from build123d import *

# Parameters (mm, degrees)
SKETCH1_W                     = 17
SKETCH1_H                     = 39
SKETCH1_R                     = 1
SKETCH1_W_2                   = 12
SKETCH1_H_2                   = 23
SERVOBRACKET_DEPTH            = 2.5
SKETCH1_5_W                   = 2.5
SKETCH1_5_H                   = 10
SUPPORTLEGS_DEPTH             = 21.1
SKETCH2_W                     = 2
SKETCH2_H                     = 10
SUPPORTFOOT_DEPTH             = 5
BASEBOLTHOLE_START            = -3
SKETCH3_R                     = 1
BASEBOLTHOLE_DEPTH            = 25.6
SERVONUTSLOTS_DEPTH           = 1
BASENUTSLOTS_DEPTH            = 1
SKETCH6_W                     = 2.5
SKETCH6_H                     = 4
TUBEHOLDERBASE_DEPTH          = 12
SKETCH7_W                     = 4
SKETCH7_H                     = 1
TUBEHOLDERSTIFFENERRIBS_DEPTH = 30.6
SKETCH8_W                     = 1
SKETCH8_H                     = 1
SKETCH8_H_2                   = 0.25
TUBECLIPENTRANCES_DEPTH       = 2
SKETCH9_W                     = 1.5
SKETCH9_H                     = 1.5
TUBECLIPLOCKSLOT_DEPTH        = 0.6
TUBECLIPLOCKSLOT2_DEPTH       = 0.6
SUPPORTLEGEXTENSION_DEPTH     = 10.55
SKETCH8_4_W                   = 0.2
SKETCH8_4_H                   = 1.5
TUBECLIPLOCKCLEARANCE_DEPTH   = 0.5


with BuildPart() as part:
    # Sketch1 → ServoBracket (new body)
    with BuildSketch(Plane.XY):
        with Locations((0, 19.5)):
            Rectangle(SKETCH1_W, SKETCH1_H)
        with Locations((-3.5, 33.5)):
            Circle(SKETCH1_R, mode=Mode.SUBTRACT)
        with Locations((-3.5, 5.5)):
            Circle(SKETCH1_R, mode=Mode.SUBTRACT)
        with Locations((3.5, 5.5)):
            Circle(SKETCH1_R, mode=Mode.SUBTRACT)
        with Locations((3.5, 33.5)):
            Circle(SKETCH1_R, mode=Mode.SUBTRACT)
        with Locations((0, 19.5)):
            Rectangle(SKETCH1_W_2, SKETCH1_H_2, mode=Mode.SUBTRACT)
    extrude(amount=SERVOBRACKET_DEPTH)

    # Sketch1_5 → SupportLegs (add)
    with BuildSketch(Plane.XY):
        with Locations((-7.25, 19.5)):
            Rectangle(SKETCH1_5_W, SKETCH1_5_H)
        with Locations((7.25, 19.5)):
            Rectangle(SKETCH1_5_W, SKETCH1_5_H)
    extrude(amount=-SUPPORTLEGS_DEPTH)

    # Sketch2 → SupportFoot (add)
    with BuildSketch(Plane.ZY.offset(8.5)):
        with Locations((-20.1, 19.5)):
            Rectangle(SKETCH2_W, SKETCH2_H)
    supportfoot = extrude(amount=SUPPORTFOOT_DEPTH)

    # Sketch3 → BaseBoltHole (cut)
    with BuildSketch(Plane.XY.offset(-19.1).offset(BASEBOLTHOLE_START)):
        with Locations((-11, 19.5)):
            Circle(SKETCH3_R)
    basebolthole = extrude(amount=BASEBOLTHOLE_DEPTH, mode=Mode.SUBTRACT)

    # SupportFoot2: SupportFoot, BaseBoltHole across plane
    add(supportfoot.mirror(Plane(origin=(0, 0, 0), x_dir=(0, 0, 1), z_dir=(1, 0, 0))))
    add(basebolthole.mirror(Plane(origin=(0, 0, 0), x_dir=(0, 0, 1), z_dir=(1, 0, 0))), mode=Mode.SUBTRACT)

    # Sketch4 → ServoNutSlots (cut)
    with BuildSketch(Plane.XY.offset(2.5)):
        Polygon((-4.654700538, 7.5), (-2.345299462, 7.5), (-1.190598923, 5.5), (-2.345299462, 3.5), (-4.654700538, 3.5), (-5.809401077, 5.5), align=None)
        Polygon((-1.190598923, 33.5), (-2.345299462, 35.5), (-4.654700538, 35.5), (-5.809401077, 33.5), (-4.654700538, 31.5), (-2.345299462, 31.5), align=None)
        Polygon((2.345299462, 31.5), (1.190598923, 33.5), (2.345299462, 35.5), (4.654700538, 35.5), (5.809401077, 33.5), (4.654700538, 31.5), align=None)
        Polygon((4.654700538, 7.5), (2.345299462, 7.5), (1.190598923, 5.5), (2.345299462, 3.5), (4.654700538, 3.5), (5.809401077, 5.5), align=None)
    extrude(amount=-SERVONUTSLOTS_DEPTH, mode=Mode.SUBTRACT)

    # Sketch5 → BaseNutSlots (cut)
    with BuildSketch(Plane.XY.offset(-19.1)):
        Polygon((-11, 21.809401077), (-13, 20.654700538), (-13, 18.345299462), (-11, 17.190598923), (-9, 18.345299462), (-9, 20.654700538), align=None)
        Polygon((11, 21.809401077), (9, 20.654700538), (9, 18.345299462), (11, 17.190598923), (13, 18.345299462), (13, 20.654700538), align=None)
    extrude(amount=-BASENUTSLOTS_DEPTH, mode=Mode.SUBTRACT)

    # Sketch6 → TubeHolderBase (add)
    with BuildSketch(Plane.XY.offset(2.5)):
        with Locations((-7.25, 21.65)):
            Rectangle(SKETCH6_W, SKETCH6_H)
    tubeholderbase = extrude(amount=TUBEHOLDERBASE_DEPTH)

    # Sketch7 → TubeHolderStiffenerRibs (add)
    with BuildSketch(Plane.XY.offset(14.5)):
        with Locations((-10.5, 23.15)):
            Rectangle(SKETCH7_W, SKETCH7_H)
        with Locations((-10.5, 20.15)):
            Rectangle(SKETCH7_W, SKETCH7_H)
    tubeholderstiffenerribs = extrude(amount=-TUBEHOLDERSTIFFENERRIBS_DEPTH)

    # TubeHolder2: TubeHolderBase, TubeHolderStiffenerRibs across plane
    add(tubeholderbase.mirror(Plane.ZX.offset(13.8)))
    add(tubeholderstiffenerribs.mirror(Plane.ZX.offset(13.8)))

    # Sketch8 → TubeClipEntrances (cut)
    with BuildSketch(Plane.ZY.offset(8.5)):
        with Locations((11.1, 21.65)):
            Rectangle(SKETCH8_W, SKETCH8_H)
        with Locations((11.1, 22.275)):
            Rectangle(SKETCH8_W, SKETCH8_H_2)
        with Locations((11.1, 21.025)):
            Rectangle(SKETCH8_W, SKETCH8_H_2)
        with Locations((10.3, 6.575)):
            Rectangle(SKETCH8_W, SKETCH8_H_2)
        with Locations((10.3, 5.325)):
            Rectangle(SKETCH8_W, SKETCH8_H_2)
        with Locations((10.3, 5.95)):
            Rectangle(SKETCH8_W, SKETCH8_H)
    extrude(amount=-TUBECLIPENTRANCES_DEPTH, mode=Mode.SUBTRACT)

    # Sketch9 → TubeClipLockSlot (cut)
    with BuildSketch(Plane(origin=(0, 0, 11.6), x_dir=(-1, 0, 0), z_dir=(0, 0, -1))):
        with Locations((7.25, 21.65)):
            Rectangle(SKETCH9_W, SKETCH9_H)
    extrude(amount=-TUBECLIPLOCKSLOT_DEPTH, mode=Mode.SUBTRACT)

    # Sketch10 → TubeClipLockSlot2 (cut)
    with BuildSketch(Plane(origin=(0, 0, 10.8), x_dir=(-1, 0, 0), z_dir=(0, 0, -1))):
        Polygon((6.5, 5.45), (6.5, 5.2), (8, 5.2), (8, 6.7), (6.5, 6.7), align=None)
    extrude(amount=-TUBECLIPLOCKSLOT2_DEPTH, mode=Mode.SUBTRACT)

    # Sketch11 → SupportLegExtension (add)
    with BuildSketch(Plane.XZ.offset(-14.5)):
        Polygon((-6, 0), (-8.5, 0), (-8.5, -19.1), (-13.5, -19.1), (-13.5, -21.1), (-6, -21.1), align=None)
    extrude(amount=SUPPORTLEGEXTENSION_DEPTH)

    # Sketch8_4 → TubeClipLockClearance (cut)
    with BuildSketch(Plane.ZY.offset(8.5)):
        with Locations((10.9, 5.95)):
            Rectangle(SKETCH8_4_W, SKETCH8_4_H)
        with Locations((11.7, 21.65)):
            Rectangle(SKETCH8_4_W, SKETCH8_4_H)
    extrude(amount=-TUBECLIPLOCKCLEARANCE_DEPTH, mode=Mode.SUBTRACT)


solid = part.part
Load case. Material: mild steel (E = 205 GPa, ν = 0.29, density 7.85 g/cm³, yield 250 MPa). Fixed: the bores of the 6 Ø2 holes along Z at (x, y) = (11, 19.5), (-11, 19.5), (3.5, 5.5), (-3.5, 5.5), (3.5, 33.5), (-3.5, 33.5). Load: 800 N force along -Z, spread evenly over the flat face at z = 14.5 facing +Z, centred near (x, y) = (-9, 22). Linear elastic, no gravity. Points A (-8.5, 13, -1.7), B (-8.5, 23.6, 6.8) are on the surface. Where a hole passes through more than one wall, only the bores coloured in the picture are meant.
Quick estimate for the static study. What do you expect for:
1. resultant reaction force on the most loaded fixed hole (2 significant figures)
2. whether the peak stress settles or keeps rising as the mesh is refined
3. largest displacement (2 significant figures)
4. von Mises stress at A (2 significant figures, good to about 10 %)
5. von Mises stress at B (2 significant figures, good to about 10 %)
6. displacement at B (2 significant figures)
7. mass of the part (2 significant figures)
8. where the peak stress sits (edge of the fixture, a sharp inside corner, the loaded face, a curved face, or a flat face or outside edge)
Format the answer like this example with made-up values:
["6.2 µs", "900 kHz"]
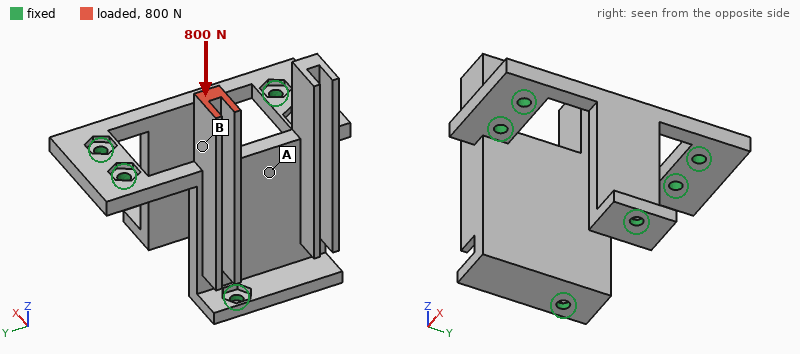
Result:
["480 N", "keeps rising", "20 µm", "21 MPa", "44 MPa", "13 µm", "27 g", "edge of the fixture"]
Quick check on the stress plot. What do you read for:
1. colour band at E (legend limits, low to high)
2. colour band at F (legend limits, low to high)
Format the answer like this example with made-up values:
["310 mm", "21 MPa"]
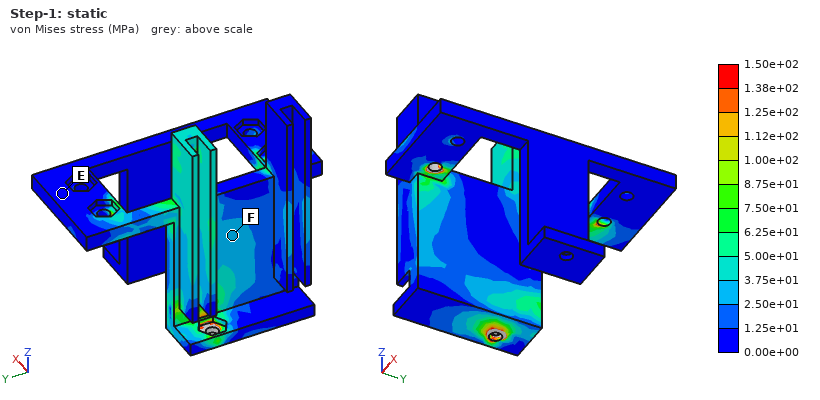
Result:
["0.00e+00 to 1.25e+01 MPa", "2.50e+01 to 3.75e+01 MPa"]
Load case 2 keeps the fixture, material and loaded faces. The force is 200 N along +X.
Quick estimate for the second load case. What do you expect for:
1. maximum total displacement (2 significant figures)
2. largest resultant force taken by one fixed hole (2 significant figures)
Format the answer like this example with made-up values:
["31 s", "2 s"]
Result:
["73 µm", "200 N"]
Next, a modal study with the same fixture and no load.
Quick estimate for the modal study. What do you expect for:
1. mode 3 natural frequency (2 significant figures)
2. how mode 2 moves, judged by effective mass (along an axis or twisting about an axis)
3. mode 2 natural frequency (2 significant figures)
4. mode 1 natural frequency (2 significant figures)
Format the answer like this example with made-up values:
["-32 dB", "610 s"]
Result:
["10 kHz", "along X", "8300 Hz", "7800 Hz"]
